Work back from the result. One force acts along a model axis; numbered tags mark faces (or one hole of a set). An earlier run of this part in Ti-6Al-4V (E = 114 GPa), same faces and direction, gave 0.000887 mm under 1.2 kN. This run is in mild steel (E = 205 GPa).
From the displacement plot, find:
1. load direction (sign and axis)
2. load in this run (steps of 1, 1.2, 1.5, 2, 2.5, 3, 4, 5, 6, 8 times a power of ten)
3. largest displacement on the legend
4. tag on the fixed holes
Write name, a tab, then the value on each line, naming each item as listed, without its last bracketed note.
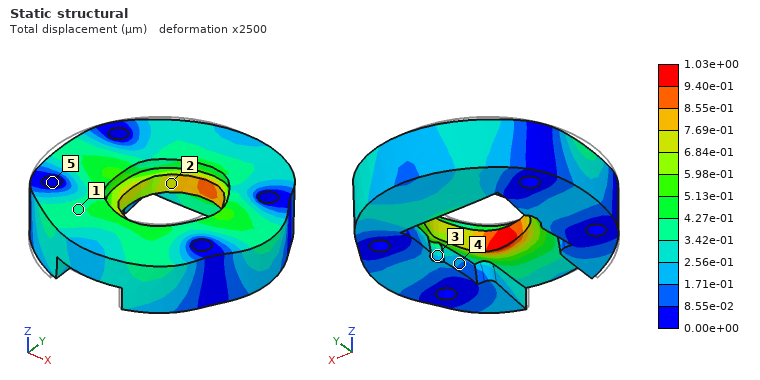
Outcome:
load direction	+X
load in this run	2.5 kN
largest displacement on the legend	1.03e+00 µm
tag on the fixed holes	5
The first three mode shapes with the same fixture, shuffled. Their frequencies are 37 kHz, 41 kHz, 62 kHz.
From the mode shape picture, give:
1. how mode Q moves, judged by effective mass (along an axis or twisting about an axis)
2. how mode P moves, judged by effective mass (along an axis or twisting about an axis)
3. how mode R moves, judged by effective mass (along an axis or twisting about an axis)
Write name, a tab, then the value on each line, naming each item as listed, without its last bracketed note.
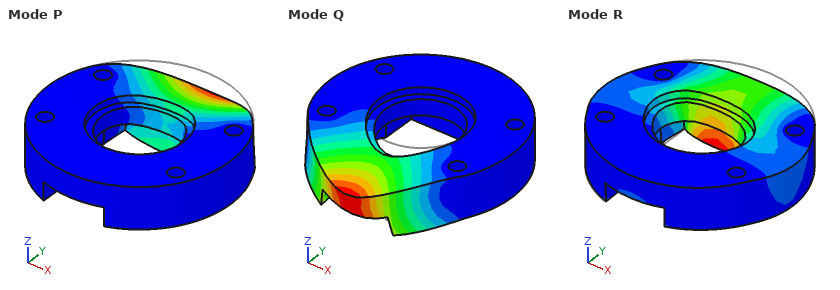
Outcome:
how mode Q moves, judged by effective mass	along Z
how mode P moves, judged by effective mass	along Z
how mode R moves, judged by effective mass	along Y
